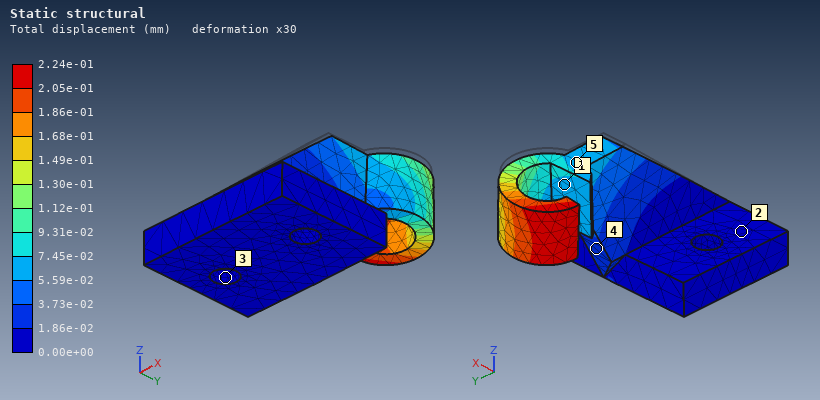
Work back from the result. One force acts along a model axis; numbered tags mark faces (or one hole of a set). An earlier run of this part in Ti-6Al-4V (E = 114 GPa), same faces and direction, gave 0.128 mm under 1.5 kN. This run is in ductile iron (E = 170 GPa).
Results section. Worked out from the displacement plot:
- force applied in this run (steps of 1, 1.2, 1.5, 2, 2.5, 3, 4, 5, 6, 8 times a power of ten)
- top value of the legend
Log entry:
4 kN
2.24e-01 mm
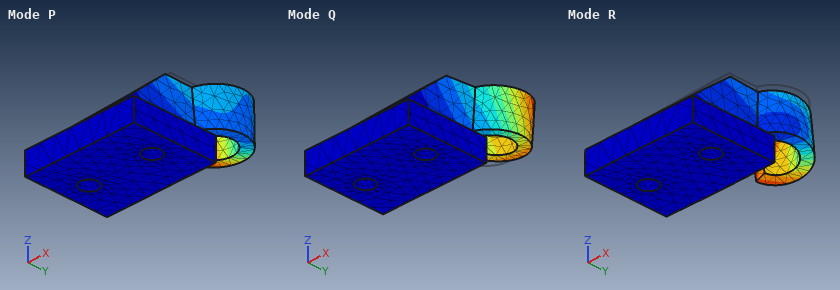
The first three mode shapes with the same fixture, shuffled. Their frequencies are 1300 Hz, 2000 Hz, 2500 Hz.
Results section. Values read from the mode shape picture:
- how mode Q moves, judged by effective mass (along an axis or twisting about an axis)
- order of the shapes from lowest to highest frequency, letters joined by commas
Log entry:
along X
Q, R, P
